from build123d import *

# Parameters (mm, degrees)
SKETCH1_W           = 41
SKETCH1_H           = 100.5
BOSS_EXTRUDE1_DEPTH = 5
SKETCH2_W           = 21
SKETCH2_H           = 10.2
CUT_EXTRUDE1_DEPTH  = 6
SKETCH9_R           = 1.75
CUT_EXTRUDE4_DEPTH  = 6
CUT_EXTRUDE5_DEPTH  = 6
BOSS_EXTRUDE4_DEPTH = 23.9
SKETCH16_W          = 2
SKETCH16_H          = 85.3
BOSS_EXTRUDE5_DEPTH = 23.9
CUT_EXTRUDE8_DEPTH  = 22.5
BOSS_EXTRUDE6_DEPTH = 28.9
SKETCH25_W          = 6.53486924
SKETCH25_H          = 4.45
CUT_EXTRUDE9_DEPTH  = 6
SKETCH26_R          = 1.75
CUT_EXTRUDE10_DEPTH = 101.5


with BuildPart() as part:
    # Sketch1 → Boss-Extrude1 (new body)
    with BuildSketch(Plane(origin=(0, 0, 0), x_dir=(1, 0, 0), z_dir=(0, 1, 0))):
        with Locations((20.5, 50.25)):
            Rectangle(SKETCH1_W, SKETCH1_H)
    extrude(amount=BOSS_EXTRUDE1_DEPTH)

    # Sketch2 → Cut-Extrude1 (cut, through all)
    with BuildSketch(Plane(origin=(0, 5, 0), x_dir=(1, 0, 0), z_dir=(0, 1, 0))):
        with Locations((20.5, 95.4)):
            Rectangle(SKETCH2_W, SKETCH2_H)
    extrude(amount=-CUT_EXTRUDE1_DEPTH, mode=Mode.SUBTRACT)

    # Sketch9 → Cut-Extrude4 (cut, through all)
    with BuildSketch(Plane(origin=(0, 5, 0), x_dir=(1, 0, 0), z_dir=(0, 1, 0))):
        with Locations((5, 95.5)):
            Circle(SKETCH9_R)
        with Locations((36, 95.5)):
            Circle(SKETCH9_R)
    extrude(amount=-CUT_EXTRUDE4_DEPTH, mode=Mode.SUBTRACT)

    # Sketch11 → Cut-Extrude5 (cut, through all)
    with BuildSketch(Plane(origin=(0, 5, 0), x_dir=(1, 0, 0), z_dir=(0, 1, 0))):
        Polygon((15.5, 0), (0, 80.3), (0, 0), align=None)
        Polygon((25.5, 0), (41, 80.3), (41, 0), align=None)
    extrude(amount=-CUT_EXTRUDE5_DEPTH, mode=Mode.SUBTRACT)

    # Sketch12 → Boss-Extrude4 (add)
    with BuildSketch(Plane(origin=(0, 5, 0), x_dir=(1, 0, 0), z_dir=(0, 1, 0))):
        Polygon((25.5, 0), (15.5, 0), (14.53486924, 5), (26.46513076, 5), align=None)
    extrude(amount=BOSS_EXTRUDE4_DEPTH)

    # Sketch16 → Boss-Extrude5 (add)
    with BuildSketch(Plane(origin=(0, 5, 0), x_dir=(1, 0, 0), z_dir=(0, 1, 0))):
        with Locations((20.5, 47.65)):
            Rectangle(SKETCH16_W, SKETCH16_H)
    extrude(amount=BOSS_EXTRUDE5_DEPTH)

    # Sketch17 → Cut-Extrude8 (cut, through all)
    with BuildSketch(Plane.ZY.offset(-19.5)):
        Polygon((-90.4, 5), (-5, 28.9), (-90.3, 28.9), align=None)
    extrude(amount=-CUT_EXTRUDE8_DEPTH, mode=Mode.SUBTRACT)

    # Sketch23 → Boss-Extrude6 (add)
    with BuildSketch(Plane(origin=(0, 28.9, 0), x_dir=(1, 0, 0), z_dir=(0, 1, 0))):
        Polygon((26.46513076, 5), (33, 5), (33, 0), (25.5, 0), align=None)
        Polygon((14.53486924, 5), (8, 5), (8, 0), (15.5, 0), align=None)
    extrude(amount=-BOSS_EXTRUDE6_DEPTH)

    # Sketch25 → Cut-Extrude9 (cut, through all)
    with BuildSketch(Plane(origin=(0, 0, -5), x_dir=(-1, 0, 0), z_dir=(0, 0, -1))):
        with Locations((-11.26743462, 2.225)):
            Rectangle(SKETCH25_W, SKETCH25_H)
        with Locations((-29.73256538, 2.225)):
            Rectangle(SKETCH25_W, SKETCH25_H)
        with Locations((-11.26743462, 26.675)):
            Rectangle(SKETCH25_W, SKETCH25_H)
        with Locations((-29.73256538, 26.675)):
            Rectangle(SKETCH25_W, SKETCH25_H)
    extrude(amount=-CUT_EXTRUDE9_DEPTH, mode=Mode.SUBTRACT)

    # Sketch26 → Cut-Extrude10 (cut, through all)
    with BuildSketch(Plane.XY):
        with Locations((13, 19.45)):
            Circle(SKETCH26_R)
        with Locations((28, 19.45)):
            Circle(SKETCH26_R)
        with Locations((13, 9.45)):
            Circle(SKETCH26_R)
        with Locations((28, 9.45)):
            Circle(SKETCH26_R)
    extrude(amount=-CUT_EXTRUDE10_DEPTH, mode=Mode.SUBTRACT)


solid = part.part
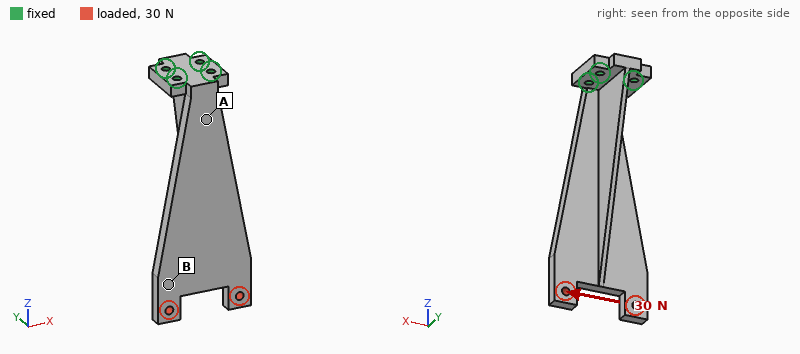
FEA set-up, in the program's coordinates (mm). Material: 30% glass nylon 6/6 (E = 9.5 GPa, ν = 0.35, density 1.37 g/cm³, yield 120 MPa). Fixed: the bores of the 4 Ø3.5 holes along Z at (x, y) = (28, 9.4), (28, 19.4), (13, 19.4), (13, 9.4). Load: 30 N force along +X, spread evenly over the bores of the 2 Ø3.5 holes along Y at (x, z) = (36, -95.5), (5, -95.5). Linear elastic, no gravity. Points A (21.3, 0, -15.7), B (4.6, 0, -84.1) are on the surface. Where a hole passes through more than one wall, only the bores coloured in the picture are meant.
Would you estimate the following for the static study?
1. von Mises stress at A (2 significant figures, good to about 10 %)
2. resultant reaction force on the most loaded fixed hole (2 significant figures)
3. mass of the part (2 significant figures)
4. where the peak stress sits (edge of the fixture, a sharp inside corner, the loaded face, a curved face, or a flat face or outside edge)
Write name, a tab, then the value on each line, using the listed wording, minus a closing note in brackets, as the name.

von Mises stress at A	3.6 MPa
resultant reaction force on the most loaded fixed hole	210 N
mass of the part	24 g
where the peak stress sits	a flat face or outside edge
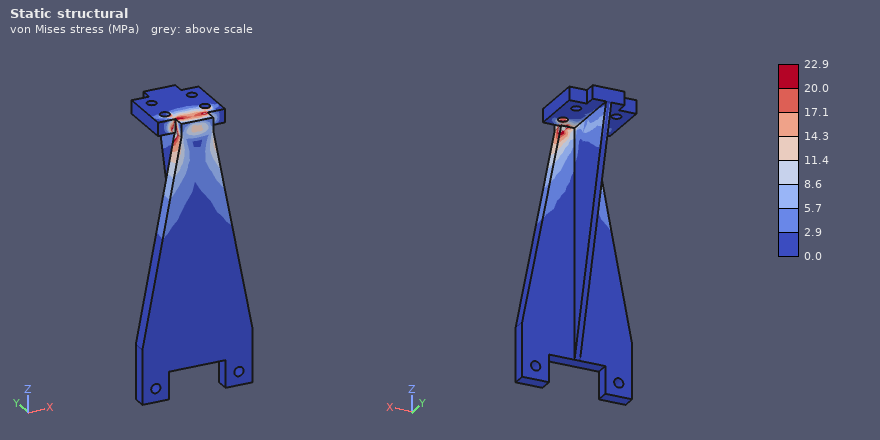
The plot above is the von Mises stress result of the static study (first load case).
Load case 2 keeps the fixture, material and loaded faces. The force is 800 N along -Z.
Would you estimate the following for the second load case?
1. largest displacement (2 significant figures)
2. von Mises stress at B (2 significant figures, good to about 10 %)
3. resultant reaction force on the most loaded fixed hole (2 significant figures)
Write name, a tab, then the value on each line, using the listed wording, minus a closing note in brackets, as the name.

largest displacement	0.56 mm
von Mises stress at B	7.4 MPa
resultant reaction force on the most loaded fixed hole	500 N
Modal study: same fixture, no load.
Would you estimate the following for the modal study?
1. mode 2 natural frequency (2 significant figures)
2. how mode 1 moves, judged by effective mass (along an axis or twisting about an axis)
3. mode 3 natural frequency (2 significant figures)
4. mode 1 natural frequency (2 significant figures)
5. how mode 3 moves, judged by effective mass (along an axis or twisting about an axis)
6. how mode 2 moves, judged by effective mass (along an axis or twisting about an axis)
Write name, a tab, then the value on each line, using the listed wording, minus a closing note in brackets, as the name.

mode 2 natural frequency	610 Hz
how mode 1 moves, judged by effective mass	along X
mode 3 natural frequency	840 Hz
mode 1 natural frequency	360 Hz
how mode 3 moves, judged by effective mass	twisting about Z
how mode 2 moves, judged by effective mass	along Y
